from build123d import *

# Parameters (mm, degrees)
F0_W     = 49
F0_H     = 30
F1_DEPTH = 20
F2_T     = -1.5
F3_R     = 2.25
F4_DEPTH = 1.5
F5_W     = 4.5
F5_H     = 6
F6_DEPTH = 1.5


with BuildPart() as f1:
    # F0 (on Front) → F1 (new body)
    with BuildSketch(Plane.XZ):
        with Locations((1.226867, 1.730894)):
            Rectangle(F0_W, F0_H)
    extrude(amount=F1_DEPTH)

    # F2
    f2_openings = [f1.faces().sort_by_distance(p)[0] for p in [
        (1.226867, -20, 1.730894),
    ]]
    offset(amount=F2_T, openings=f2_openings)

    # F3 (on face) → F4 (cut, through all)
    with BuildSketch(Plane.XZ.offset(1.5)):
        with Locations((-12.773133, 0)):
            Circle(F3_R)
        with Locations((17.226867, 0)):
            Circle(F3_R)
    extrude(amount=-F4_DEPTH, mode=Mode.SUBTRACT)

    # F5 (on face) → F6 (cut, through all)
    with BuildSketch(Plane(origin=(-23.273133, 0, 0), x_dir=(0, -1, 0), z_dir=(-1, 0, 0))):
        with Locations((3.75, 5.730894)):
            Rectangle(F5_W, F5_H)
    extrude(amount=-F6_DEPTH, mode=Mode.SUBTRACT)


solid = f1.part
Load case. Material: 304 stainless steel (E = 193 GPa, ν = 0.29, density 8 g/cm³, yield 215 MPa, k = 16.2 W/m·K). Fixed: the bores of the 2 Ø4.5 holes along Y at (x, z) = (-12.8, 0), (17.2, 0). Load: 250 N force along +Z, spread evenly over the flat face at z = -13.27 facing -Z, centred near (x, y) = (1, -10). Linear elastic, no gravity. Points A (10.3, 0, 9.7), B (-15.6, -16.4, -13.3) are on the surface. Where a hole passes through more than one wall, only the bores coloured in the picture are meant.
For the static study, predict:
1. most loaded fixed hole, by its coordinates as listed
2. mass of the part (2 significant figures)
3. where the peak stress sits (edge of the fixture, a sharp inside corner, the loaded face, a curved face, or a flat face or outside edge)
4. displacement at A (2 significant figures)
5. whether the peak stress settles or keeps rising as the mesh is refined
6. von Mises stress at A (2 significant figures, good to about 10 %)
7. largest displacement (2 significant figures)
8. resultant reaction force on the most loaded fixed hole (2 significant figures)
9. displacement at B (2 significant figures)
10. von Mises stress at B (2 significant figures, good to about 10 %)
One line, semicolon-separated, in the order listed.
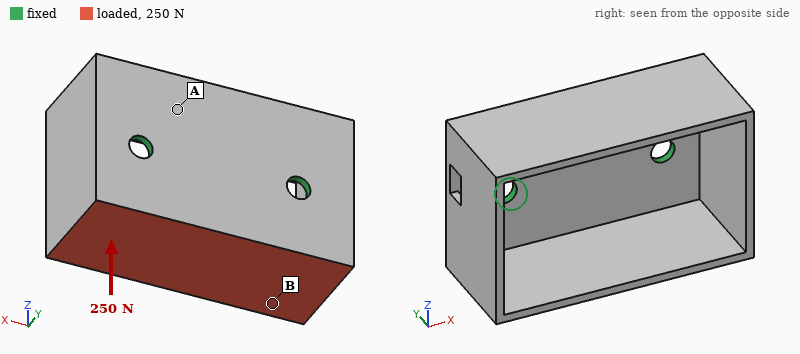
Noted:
(-12.8, 0); 51 g; edge of the fixture; 14 µm; keeps rising; 16 MPa; 92 µm; 140 N; 54 µm; 32 MPa
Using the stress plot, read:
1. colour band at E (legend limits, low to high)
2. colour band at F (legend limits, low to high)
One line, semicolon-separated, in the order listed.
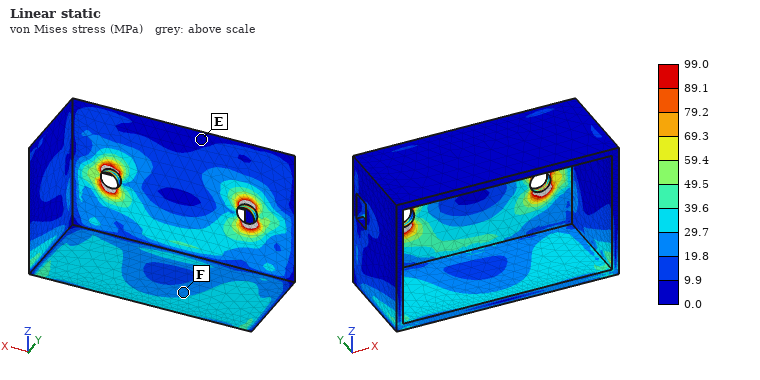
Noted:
0.0 to 9.9 MPa; 19.8 to 29.7 MPa
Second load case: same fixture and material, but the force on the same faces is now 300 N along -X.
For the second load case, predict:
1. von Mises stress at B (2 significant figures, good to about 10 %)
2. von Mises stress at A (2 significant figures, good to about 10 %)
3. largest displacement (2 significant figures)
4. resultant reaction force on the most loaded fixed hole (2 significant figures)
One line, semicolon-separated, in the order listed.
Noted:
9.6 MPa; 6.0 MPa; 28 µm; 210 N
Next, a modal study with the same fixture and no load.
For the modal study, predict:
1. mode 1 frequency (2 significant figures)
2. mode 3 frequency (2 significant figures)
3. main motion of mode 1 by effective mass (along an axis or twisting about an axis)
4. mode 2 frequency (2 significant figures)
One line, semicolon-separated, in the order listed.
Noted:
1700 Hz; 3900 Hz; along Z; 2400 Hz
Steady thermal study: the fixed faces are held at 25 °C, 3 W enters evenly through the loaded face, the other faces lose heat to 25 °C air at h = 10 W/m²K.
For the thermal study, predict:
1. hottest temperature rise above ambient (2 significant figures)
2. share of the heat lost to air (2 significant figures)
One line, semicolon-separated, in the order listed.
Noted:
37 K; 31 %
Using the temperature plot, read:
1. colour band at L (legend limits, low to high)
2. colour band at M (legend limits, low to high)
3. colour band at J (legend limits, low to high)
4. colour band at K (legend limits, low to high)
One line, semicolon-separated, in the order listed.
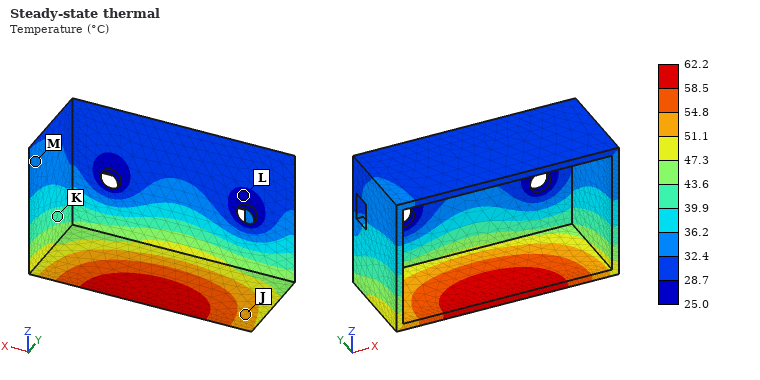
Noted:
25.0 to 28.7 °C; 32.4 to 36.2 °C; 51.1 to 54.8 °C; 39.9 to 43.6 °C
